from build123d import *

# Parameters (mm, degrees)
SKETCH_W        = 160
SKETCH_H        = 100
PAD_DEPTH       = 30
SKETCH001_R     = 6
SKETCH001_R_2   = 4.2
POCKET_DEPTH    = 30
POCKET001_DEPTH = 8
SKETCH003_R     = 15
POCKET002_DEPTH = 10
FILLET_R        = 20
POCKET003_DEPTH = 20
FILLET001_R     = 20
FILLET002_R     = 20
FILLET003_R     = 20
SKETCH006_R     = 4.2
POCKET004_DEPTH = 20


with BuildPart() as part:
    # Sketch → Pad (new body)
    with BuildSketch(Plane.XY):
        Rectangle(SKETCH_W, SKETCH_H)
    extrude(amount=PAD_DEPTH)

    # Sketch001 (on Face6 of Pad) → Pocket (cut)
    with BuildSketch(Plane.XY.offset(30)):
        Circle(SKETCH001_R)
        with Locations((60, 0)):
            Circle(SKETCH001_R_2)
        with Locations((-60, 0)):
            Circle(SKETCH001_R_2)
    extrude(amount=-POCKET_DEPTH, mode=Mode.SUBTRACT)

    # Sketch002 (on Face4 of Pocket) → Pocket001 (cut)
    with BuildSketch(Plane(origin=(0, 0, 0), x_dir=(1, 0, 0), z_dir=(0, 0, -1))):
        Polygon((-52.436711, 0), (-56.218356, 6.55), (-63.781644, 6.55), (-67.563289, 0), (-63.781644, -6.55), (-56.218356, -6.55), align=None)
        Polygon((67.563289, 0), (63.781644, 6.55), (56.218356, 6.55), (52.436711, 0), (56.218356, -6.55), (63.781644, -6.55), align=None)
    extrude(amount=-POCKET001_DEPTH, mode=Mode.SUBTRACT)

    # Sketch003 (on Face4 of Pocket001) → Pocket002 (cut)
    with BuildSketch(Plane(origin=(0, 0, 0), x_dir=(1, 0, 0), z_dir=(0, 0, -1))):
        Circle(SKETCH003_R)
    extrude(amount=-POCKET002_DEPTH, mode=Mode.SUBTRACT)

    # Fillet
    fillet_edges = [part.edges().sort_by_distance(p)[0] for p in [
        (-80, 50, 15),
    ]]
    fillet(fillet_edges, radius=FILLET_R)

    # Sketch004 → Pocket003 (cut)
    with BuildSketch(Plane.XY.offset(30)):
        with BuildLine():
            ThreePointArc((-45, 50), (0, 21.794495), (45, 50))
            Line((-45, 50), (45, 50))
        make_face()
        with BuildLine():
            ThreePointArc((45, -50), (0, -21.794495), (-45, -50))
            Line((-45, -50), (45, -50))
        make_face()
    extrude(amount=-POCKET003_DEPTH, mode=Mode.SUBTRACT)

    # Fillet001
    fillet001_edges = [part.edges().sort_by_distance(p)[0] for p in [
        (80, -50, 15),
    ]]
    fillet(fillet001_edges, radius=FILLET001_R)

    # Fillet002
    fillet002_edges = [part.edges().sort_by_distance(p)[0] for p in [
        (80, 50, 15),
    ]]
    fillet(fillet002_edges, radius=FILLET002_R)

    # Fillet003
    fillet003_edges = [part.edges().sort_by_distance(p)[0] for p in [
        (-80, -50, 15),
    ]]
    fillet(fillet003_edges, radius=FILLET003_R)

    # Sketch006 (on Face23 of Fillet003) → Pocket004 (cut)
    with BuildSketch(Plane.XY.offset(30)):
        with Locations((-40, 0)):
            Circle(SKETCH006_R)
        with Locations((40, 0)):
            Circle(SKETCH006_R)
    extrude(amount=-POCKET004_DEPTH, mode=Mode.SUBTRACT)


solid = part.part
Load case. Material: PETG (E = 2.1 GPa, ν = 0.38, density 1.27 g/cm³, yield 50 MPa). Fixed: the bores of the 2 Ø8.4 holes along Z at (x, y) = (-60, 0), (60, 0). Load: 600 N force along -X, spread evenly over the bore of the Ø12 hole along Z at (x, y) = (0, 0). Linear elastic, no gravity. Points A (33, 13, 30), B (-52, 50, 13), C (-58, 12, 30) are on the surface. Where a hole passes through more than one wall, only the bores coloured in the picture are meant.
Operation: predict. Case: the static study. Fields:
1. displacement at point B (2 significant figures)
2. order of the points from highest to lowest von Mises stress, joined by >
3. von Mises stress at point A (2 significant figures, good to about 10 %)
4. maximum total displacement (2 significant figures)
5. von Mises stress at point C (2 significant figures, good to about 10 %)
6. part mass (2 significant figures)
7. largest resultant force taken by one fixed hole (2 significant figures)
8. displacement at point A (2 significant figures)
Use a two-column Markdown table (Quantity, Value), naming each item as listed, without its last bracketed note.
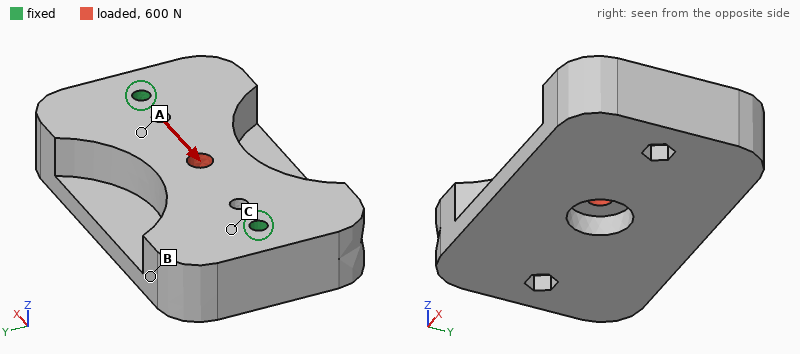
| Quantity | Value |
|---|---|
| displacement at point B | 6.0 µm |
| order of the points from highest to lowest von Mises stress, joined by > | A > C > B |
| von Mises stress at point A | 0.37 MPa |
| maximum total displacement | 13 µm |
| von Mises stress at point C | 0.18 MPa |
| part mass | 480 g |
| largest resultant force taken by one fixed hole | 300 N |
| displacement at point A | 5.5 µm |
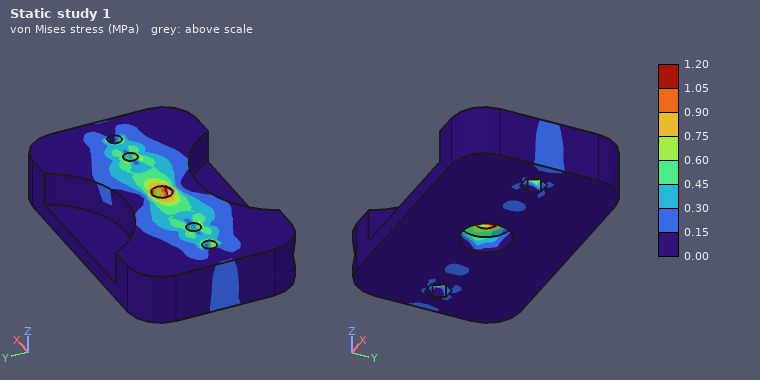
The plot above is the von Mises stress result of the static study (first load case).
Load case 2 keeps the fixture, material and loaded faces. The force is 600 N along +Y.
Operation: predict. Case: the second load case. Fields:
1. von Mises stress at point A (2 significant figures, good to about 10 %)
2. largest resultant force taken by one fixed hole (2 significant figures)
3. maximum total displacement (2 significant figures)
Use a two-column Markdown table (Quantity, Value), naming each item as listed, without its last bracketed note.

| Quantity | Value |
|---|---|
| von Mises stress at point A | 0.32 MPa |
| largest resultant force taken by one fixed hole | 300 N |
| maximum total displacement | 32 µm |
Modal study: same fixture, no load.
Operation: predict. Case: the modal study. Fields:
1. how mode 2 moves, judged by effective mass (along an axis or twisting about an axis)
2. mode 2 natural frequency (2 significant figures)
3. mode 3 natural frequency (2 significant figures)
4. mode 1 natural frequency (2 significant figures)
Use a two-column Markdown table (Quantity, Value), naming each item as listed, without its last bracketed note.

| Quantity | Value |
|---|---|
| how mode 2 moves, judged by effective mass | along Z |
| mode 2 natural frequency | 1300 Hz |
| mode 3 natural frequency | 1400 Hz |
| mode 1 natural frequency | 990 Hz |
